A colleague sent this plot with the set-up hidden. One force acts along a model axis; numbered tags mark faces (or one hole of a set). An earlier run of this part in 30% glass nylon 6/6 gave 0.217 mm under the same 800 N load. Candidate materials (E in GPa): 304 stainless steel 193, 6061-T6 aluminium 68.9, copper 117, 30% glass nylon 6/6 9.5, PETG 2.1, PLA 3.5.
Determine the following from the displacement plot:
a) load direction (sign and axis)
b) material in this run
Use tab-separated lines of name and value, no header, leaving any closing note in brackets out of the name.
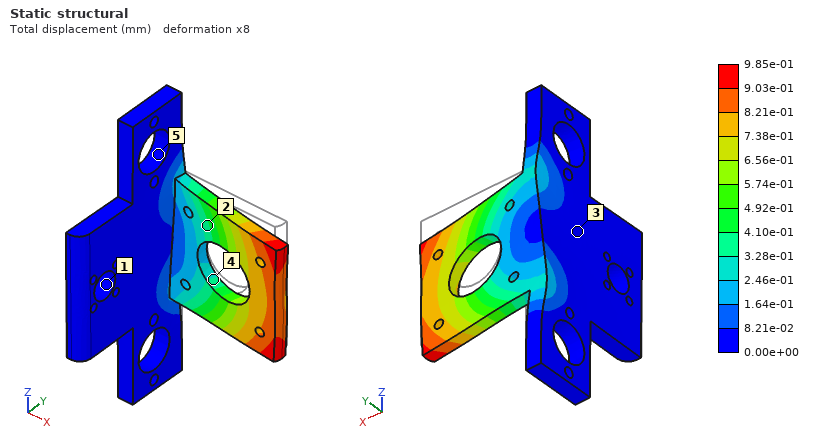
load direction	-Z
material in this run	PETG
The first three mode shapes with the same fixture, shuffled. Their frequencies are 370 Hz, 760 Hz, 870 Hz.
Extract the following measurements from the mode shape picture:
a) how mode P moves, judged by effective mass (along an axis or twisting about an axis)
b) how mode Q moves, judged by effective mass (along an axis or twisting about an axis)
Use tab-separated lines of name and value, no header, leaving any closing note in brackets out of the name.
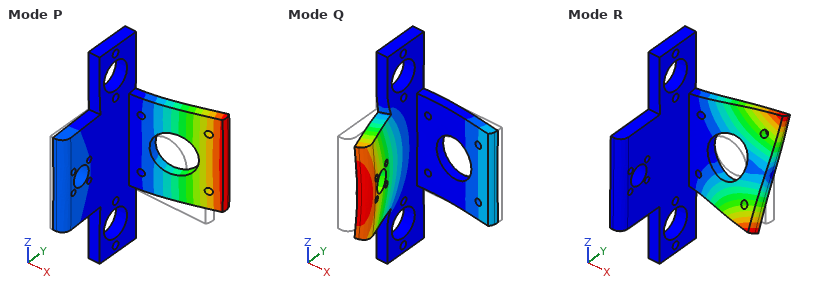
how mode P moves, judged by effective mass	along Y
how mode Q moves, judged by effective mass	along X
